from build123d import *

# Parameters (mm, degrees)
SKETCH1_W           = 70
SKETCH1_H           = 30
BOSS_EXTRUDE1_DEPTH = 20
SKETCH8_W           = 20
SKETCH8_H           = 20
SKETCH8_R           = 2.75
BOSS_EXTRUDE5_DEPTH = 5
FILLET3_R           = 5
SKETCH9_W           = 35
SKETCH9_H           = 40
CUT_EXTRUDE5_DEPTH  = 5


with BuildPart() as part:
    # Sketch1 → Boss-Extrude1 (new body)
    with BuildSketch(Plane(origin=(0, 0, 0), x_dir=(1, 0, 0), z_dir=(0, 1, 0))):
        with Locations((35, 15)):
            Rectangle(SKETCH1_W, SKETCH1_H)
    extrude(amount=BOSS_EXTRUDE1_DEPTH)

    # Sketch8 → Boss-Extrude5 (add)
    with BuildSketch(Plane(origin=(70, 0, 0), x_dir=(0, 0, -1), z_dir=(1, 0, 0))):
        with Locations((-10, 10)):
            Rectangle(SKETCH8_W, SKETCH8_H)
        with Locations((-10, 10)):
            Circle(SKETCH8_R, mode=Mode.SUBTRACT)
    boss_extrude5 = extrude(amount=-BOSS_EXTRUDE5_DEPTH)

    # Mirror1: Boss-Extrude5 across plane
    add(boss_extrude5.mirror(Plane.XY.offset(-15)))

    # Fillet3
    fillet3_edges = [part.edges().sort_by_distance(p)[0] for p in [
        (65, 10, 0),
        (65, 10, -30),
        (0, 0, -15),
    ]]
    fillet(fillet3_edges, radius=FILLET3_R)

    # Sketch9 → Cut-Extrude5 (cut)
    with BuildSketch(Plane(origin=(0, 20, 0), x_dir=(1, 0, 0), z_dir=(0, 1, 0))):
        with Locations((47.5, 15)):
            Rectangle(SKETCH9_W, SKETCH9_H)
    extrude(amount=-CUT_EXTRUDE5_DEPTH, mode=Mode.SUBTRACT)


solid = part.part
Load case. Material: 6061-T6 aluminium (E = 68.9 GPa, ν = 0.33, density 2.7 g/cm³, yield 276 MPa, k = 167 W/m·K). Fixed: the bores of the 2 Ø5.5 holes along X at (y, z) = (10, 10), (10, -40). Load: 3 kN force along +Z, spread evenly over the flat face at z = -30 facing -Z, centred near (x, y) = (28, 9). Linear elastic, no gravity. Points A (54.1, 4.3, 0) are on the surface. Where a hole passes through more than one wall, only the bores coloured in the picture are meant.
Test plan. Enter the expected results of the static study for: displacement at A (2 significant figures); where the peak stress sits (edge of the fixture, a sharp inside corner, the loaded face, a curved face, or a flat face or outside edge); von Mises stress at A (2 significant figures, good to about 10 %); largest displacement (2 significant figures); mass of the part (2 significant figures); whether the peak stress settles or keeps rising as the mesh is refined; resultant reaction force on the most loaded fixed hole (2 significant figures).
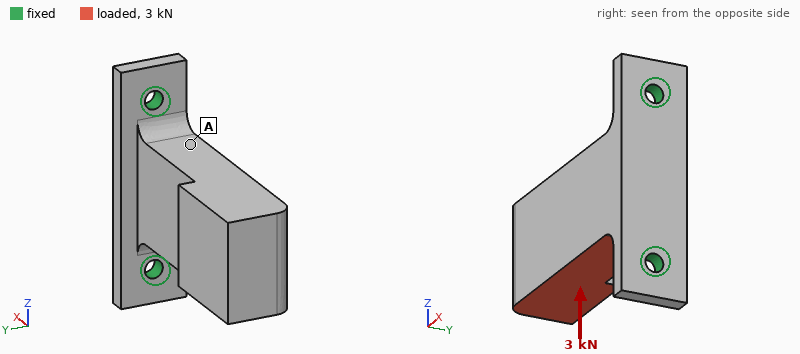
0.041 mm
edge of the fixture
35 MPa
0.18 mm
110 g
keeps rising
3.3 kN
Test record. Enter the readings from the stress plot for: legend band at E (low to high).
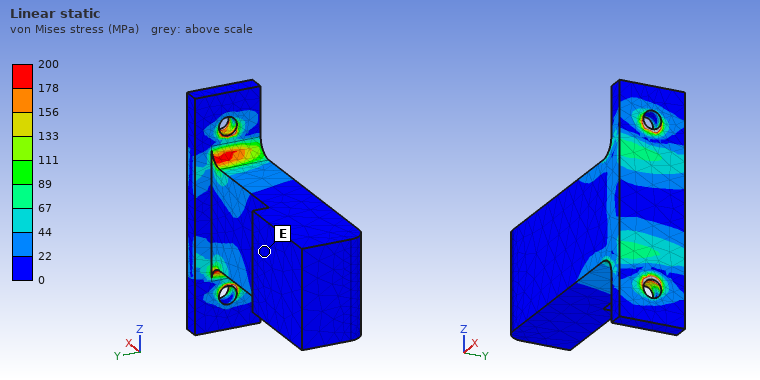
0 to 22 MPa
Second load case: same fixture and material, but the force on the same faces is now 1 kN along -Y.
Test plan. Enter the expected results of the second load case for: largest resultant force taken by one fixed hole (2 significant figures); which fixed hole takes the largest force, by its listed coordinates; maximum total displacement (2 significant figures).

820 N
(10, -40)
0.61 mm
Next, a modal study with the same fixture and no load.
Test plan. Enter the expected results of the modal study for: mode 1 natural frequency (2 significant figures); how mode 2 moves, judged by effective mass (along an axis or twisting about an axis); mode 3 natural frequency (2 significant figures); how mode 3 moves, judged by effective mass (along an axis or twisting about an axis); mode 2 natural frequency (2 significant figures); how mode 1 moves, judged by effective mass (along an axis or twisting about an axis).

850 Hz
along Z
6000 Hz
along X
2700 Hz
along Y
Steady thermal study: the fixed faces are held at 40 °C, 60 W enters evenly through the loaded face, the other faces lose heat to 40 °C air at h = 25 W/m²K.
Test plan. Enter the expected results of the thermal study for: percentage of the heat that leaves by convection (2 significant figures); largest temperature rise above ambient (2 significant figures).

10 %
49 K
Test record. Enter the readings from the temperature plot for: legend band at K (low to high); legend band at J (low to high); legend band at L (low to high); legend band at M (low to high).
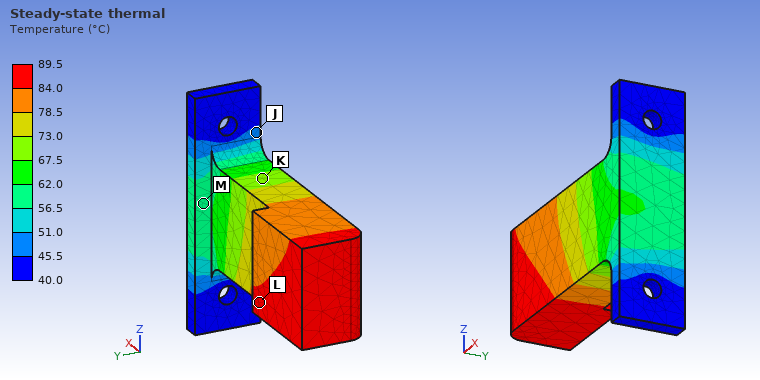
67.5 to 73.0 °C
45.5 to 51.0 °C
84.0 to 89.5 °C
56.5 to 62.0 °C
